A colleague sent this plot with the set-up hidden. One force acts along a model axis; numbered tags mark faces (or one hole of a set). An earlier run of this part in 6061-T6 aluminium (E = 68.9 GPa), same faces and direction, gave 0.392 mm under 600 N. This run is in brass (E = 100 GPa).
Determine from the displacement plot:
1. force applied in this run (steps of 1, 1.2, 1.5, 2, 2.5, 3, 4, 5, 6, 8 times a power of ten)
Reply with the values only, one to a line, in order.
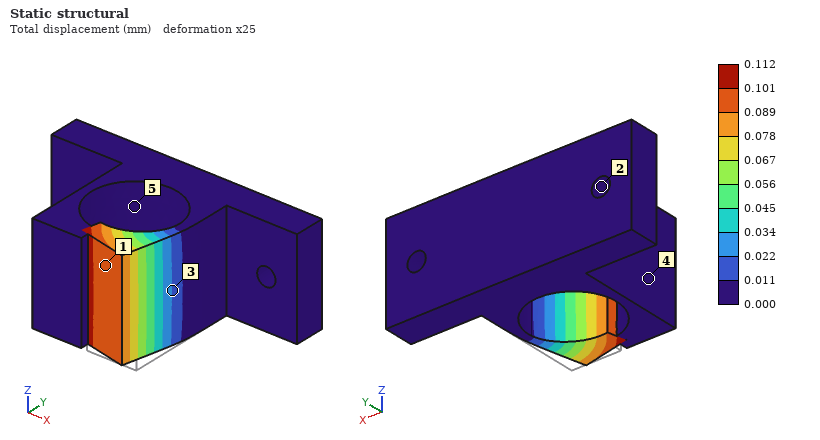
250 N
